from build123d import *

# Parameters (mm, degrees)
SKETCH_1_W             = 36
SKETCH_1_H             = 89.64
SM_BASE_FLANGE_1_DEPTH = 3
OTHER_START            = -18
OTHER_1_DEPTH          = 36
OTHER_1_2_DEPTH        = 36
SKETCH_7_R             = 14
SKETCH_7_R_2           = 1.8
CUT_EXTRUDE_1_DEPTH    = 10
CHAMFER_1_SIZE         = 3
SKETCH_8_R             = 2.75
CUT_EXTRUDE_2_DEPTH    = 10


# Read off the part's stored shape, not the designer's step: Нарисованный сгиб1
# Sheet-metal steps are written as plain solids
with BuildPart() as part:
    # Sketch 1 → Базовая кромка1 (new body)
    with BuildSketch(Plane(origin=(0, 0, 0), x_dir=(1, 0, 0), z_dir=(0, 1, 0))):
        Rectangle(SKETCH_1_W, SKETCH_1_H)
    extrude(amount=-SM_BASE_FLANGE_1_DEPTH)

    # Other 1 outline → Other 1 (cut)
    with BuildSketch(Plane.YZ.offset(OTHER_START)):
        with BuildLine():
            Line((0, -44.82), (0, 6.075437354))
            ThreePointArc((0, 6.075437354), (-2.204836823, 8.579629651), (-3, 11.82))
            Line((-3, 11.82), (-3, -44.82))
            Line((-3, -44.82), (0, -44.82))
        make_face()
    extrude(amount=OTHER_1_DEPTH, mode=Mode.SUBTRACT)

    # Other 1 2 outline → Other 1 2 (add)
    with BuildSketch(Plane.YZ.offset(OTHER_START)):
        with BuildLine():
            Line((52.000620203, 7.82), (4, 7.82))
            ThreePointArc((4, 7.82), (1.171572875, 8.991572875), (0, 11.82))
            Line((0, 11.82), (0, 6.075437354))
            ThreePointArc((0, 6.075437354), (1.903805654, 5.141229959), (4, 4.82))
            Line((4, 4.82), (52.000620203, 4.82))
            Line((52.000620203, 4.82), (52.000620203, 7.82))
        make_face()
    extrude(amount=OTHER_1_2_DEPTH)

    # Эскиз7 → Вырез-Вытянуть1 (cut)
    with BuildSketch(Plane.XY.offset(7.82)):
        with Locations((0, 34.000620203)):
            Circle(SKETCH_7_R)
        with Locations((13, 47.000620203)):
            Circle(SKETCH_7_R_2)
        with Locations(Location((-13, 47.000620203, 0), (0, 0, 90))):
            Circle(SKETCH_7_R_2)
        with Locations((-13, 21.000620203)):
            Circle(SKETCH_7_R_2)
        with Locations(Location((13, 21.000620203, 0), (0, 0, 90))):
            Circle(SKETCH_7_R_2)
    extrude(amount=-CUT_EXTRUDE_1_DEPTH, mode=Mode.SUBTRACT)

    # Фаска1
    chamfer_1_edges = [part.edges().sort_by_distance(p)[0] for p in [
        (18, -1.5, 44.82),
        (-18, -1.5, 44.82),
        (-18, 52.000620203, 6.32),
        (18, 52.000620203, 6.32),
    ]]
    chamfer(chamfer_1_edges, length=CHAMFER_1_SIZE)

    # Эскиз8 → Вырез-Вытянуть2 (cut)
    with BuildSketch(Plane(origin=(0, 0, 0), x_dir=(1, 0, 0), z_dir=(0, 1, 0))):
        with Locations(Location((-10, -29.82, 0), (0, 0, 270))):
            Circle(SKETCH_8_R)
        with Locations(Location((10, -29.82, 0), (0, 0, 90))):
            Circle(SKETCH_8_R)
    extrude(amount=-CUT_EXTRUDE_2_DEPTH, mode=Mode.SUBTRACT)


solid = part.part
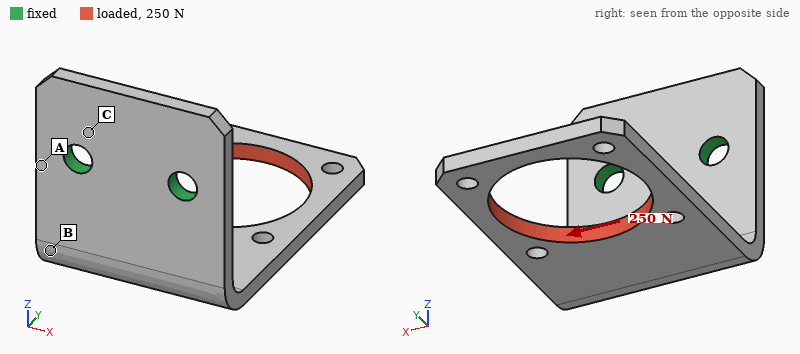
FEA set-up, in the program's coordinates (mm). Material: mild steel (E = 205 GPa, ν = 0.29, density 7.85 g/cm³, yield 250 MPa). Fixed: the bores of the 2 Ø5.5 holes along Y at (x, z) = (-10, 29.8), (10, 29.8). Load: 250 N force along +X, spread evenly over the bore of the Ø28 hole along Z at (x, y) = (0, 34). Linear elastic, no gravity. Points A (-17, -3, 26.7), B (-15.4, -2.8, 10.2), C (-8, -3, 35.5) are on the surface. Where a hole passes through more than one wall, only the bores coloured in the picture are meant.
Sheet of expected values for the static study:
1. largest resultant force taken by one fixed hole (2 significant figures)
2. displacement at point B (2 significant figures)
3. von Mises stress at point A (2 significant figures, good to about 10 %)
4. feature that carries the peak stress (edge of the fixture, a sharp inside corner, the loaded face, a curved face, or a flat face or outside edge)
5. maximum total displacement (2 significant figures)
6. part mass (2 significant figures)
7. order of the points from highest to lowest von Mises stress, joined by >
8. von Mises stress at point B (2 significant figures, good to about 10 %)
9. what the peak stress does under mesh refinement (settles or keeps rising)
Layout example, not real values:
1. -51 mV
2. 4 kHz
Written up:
1. 450 N
2. 0.050 mm
3. 100 MPa
4. edge of the fixture
5. 0.23 mm
6. 59 g
7. A > B > C
8. 70 MPa
9. keeps rising
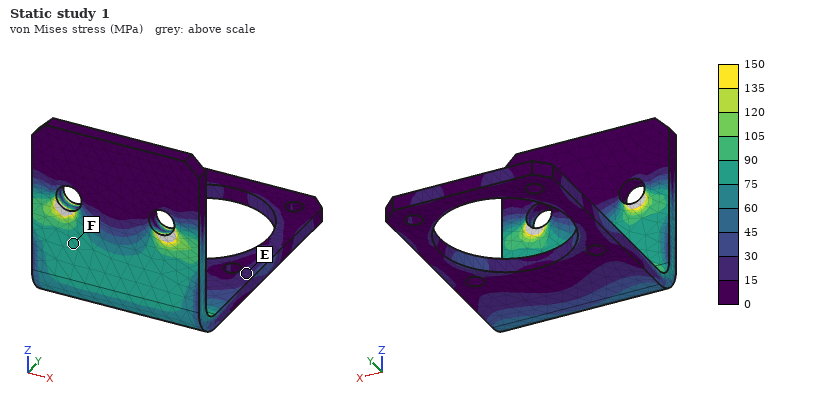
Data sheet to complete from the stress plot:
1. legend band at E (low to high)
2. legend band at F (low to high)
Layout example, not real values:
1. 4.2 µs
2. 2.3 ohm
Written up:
1. 15 to 30 MPa
2. 75 to 90 MPa
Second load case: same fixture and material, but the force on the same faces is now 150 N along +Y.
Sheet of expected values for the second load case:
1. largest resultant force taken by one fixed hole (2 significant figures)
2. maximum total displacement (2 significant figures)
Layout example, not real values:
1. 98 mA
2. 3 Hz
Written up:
1. 75 N
2. 0.12 mm
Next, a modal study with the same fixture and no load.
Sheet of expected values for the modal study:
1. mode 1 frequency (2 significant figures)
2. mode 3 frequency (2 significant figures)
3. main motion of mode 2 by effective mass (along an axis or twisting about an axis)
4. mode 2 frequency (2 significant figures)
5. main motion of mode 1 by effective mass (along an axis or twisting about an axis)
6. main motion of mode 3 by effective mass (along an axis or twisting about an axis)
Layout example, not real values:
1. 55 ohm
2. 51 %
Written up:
1. 700 Hz
2. 2300 Hz
3. along X
4. 1400 Hz
5. along Z
6. along Y
